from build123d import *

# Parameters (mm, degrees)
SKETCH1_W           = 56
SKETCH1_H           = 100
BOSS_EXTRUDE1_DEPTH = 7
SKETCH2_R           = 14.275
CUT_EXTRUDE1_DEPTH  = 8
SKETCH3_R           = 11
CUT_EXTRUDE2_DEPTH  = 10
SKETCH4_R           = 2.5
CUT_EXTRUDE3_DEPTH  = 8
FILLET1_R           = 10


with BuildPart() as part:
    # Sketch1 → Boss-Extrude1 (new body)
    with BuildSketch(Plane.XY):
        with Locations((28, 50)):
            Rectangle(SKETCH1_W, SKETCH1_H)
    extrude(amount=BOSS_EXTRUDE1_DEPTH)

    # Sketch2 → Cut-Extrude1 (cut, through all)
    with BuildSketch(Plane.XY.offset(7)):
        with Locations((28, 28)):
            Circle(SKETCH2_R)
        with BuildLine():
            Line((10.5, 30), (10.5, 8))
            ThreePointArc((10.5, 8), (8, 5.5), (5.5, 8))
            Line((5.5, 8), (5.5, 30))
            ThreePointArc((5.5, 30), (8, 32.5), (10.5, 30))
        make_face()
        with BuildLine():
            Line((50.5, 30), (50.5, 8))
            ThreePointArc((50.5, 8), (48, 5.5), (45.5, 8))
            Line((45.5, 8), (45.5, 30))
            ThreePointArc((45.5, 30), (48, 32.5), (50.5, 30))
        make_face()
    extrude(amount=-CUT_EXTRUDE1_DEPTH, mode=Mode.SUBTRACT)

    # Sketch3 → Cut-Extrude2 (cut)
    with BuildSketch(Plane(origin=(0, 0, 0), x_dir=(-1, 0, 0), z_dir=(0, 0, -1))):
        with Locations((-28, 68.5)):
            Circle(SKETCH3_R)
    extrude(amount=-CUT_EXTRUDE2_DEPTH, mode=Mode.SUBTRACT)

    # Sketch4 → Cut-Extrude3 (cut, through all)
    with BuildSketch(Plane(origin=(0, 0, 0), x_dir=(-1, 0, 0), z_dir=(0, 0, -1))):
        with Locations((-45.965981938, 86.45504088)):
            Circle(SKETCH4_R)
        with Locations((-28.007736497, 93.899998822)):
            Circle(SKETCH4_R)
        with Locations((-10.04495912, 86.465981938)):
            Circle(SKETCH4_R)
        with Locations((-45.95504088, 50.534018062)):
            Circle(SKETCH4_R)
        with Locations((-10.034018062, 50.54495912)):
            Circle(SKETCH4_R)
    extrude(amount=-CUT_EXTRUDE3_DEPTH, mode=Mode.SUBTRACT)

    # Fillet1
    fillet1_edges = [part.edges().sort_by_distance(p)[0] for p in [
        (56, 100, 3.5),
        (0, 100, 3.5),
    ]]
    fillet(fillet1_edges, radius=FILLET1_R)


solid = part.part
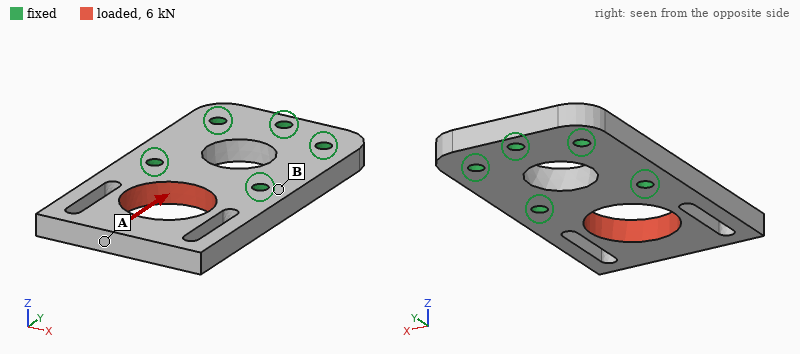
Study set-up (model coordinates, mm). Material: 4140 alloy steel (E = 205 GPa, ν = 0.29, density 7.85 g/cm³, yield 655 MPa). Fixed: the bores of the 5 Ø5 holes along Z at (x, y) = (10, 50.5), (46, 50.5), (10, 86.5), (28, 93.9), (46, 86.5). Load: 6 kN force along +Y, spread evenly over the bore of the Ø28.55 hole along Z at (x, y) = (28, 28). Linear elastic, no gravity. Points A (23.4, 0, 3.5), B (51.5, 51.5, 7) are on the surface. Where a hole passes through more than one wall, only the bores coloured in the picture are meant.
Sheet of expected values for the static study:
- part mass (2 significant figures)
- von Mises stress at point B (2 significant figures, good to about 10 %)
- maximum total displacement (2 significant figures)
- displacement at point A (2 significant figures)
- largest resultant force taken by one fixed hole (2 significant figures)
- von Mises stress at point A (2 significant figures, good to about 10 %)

230 g
9.5 MPa
8.2 µm
7.5 µm
2.8 kN
26 MPa
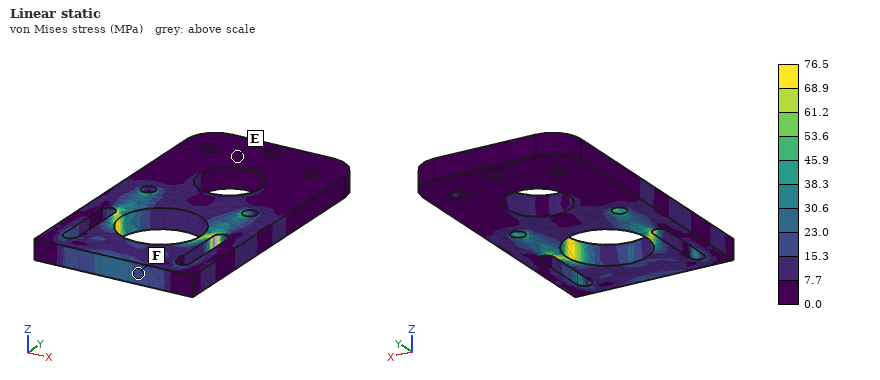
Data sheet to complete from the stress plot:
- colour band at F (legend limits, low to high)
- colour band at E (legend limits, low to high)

15.3 to 23.0 MPa
0.0 to 7.7 MPa
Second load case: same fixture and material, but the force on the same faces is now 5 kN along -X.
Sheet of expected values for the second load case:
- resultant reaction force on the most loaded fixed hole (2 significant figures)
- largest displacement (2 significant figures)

3.3 kN
54 µm
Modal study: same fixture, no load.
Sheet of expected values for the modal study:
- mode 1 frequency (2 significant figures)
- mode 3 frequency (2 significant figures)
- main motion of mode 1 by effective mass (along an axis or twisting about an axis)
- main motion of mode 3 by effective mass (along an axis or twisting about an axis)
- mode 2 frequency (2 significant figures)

1900 Hz
5000 Hz
along Z
along X
3900 Hz
